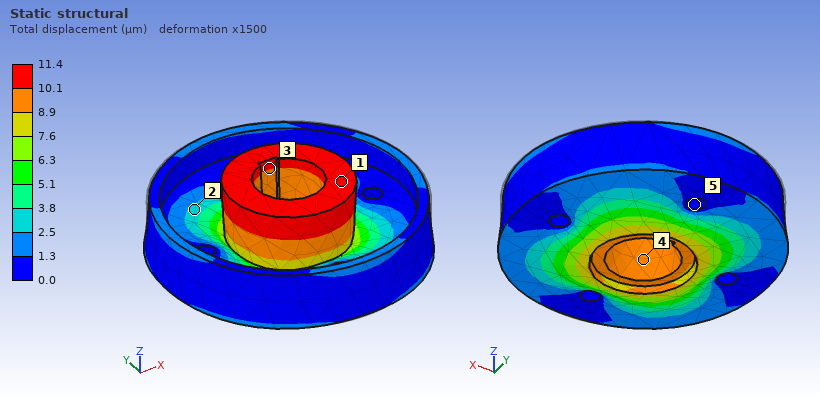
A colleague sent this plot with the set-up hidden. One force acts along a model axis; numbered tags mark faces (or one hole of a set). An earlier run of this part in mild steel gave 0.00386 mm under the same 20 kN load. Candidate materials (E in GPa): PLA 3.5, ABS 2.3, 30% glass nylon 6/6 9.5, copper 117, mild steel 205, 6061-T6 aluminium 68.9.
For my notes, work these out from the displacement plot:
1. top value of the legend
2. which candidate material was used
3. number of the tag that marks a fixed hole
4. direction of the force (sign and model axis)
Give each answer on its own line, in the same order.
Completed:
11.4 µm
6061-T6 aluminium
5
-Z
